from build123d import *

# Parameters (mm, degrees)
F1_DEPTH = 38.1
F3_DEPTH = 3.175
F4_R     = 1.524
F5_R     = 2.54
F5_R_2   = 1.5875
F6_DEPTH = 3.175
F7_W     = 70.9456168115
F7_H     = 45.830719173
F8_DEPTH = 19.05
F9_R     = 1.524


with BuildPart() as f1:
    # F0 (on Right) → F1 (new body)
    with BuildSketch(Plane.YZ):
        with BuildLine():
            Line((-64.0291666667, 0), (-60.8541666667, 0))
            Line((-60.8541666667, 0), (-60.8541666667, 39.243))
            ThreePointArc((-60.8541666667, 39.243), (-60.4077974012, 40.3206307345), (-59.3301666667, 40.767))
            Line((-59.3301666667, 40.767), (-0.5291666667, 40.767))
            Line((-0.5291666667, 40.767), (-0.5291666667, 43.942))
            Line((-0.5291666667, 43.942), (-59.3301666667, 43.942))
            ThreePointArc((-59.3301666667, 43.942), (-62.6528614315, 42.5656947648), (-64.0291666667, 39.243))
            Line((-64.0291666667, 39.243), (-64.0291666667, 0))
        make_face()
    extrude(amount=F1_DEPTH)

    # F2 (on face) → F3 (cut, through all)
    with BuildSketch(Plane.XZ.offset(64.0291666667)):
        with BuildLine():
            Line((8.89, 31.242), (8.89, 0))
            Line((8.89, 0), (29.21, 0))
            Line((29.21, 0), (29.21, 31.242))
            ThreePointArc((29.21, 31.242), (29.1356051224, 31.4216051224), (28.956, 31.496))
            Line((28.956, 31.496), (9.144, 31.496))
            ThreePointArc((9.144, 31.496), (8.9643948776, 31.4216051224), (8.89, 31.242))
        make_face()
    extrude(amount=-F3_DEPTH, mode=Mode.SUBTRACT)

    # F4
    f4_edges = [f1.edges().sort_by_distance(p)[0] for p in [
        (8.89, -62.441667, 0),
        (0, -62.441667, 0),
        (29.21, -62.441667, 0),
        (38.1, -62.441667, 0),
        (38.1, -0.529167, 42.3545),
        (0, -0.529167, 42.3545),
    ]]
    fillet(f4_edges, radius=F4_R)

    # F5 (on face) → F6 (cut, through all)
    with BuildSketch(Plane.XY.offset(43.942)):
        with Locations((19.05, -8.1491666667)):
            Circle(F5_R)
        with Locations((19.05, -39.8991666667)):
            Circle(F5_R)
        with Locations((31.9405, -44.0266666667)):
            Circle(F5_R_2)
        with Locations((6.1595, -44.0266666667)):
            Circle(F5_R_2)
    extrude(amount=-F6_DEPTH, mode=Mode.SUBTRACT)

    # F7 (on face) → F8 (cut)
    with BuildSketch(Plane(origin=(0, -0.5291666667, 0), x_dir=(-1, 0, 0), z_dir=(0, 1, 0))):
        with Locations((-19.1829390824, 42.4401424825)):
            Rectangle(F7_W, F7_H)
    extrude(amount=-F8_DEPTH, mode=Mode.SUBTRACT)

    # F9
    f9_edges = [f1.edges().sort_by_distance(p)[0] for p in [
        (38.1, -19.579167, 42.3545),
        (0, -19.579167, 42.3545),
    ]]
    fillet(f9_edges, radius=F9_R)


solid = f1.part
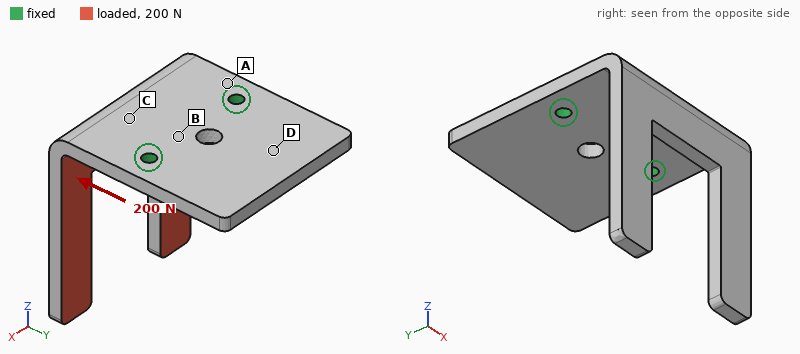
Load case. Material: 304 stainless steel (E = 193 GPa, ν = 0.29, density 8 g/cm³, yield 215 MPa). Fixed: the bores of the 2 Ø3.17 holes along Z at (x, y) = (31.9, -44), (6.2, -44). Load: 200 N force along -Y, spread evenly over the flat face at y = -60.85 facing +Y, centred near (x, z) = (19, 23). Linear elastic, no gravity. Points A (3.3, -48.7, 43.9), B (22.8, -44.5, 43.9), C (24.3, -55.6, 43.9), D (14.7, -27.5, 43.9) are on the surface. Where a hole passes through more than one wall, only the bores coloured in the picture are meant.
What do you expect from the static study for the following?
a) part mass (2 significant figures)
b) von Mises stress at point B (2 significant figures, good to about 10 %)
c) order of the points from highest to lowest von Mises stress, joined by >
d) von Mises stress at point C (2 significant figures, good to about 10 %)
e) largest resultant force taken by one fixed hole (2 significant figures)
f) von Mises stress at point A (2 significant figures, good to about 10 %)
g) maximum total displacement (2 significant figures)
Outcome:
64 g
30 MPa
A > C > B > D
52 MPa
100 N
65 MPa
0.29 mm
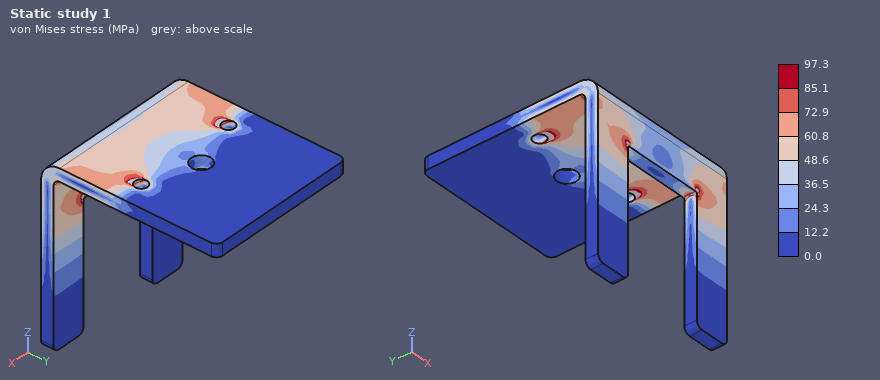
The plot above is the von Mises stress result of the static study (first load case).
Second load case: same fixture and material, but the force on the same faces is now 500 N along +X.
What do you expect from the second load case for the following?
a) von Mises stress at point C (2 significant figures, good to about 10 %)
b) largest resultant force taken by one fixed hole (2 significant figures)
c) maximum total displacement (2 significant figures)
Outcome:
65 MPa
530 N
0.18 mm
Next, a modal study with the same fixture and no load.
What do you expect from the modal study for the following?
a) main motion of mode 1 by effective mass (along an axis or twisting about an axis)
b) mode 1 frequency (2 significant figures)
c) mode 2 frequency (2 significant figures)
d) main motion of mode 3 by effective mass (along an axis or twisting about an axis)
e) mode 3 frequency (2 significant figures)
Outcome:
along Y
1100 Hz
1500 Hz
along X
2400 Hz
